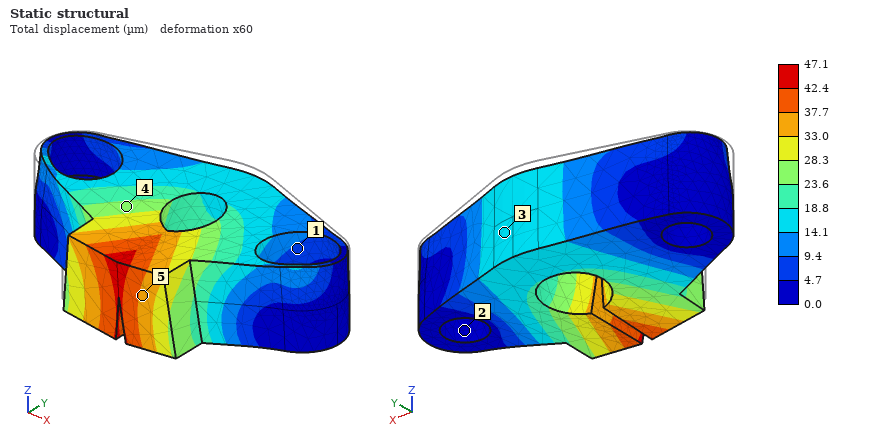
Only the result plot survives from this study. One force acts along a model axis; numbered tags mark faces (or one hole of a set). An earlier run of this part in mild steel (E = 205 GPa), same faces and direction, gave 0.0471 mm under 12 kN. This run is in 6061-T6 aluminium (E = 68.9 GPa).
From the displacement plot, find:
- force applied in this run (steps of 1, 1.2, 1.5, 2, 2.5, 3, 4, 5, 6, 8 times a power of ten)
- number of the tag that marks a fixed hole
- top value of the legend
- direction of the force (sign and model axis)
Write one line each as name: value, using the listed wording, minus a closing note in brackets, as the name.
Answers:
force applied in this run: 4 kN
number of the tag that marks a fixed hole: 2
top value of the legend: 47.1 µm
direction of the force: -Z
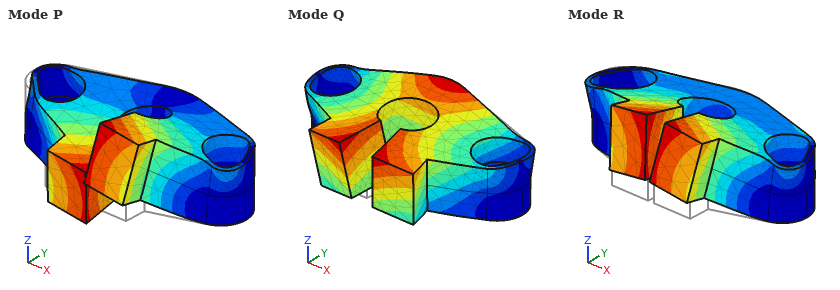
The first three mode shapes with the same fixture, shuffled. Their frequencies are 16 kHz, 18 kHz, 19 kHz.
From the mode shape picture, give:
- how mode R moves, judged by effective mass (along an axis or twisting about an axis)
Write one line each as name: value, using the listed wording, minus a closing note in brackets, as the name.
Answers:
how mode R moves, judged by effective mass: along Z
